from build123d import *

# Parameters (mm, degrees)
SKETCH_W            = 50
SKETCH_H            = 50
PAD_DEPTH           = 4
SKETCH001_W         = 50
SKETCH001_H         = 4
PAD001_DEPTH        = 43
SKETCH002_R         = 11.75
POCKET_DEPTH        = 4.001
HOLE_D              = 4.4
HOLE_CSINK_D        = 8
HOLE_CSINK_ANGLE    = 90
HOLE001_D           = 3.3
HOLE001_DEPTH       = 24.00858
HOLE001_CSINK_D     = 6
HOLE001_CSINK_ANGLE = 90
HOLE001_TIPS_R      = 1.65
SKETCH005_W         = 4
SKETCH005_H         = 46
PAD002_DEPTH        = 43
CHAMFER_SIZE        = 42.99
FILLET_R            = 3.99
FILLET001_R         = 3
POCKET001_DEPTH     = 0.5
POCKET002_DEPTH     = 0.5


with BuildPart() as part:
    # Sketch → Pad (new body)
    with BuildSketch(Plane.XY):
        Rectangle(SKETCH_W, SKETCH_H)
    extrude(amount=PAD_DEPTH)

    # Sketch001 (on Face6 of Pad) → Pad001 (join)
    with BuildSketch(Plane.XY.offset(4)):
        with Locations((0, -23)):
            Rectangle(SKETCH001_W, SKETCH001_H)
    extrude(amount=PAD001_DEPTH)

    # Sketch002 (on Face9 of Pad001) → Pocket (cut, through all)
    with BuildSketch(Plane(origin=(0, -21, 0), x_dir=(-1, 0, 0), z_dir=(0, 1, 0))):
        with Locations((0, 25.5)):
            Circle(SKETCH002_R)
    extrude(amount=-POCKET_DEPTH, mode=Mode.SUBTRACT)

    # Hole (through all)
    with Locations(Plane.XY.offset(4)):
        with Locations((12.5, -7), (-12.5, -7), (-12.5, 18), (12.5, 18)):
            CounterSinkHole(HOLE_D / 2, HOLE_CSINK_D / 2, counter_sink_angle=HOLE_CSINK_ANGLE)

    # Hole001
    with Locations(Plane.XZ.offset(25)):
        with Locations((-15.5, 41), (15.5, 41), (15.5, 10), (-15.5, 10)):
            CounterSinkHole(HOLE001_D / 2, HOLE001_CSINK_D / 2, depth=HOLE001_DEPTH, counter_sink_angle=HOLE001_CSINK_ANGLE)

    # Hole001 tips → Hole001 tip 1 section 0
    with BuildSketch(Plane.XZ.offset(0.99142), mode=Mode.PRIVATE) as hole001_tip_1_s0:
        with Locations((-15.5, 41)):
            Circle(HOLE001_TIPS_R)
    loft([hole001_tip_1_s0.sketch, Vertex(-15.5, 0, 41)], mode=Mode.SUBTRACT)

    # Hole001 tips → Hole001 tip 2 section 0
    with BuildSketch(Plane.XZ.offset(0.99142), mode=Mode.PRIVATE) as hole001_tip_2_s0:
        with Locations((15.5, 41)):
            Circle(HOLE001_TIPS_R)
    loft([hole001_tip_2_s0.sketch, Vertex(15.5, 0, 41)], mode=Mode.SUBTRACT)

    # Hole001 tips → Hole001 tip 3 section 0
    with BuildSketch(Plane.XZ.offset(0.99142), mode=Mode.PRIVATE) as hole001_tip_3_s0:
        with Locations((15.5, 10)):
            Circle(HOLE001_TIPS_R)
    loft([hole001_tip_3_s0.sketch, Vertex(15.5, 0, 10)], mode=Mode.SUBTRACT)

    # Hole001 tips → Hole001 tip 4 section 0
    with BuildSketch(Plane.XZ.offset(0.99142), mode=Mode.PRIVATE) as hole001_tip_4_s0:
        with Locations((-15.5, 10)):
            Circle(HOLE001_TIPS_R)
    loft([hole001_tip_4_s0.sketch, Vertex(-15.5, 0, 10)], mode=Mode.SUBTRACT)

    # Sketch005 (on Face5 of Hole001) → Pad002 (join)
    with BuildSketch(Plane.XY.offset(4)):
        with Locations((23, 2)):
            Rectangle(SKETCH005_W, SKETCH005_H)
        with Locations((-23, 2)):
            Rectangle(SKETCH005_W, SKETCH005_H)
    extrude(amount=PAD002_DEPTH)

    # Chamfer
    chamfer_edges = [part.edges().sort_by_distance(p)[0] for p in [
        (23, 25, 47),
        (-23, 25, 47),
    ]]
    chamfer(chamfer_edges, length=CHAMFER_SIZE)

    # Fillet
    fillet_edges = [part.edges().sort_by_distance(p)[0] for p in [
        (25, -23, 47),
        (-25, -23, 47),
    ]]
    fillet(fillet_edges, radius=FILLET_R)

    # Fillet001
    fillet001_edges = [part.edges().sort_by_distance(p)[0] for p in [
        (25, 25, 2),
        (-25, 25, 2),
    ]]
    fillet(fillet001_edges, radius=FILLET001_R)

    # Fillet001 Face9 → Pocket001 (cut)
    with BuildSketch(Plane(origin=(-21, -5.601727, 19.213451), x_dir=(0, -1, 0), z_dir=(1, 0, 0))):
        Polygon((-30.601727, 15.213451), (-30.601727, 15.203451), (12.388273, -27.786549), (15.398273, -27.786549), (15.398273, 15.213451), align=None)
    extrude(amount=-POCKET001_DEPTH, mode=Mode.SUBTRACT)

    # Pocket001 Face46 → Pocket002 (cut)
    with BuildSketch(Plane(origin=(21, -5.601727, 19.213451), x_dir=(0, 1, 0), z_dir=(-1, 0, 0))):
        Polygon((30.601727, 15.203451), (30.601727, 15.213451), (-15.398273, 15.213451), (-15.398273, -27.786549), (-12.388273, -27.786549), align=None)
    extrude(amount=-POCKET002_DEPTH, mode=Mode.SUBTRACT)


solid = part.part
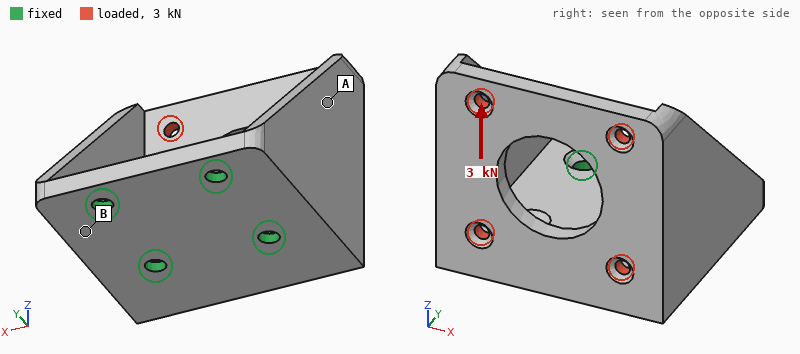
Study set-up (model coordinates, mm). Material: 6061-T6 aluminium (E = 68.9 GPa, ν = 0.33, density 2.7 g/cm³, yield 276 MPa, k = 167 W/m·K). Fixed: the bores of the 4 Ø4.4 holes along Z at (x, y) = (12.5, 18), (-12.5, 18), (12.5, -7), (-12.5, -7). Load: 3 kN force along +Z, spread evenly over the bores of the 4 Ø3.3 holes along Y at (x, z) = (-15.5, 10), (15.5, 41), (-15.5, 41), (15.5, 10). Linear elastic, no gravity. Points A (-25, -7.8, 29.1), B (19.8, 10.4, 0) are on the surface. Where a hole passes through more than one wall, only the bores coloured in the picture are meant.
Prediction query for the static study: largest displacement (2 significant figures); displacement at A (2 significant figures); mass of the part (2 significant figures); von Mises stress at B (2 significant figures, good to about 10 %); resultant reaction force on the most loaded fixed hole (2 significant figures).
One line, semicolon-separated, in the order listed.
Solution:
0.20 mm; 0.11 mm; 64 g; 44 MPa; 2.3 kN
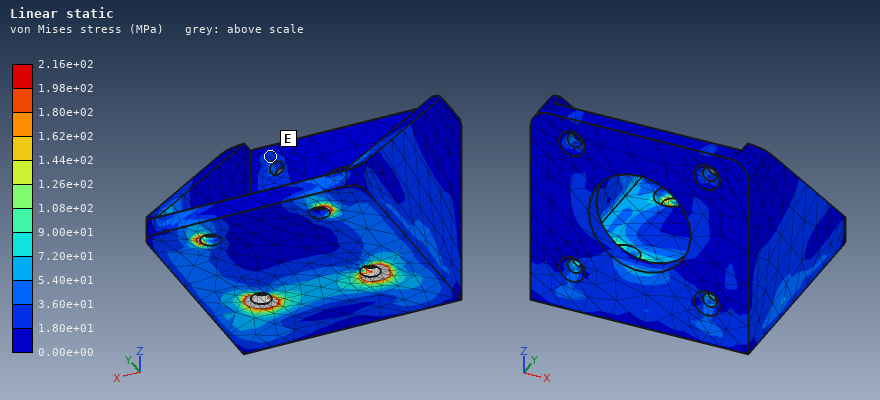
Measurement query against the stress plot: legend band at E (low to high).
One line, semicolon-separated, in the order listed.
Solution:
1.80e+01 to 3.60e+01 MPa
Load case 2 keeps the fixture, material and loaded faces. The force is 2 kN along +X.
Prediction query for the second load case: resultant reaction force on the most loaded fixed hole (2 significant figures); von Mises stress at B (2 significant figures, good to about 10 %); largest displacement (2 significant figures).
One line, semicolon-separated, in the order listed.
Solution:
2.3 kN; 47 MPa; 0.33 mm
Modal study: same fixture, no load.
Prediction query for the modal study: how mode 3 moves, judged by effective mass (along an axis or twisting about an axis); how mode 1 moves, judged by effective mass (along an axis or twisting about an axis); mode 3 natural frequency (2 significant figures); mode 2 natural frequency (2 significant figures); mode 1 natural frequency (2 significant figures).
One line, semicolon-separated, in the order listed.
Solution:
along Z; along X; 5300 Hz; 3200 Hz; 2400 Hz
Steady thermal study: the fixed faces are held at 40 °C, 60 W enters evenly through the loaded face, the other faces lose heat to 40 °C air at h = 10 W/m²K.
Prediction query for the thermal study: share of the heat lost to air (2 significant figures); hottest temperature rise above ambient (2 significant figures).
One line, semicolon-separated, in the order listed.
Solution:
4.7 %; 55 K
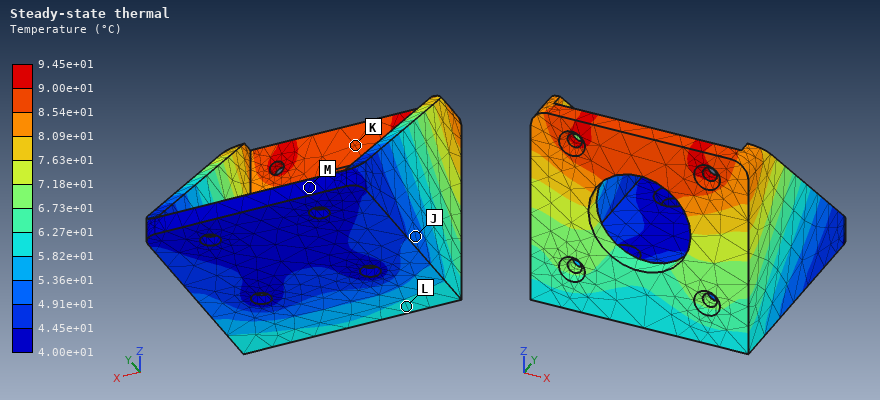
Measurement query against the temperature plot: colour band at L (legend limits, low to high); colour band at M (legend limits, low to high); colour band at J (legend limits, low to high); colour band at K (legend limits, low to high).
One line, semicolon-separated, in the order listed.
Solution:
5.82e+01 to 6.27e+01 °C; 4.00e+01 to 4.45e+01 °C; 4.91e+01 to 5.36e+01 °C; 8.54e+01 to 9.00e+01 °C
